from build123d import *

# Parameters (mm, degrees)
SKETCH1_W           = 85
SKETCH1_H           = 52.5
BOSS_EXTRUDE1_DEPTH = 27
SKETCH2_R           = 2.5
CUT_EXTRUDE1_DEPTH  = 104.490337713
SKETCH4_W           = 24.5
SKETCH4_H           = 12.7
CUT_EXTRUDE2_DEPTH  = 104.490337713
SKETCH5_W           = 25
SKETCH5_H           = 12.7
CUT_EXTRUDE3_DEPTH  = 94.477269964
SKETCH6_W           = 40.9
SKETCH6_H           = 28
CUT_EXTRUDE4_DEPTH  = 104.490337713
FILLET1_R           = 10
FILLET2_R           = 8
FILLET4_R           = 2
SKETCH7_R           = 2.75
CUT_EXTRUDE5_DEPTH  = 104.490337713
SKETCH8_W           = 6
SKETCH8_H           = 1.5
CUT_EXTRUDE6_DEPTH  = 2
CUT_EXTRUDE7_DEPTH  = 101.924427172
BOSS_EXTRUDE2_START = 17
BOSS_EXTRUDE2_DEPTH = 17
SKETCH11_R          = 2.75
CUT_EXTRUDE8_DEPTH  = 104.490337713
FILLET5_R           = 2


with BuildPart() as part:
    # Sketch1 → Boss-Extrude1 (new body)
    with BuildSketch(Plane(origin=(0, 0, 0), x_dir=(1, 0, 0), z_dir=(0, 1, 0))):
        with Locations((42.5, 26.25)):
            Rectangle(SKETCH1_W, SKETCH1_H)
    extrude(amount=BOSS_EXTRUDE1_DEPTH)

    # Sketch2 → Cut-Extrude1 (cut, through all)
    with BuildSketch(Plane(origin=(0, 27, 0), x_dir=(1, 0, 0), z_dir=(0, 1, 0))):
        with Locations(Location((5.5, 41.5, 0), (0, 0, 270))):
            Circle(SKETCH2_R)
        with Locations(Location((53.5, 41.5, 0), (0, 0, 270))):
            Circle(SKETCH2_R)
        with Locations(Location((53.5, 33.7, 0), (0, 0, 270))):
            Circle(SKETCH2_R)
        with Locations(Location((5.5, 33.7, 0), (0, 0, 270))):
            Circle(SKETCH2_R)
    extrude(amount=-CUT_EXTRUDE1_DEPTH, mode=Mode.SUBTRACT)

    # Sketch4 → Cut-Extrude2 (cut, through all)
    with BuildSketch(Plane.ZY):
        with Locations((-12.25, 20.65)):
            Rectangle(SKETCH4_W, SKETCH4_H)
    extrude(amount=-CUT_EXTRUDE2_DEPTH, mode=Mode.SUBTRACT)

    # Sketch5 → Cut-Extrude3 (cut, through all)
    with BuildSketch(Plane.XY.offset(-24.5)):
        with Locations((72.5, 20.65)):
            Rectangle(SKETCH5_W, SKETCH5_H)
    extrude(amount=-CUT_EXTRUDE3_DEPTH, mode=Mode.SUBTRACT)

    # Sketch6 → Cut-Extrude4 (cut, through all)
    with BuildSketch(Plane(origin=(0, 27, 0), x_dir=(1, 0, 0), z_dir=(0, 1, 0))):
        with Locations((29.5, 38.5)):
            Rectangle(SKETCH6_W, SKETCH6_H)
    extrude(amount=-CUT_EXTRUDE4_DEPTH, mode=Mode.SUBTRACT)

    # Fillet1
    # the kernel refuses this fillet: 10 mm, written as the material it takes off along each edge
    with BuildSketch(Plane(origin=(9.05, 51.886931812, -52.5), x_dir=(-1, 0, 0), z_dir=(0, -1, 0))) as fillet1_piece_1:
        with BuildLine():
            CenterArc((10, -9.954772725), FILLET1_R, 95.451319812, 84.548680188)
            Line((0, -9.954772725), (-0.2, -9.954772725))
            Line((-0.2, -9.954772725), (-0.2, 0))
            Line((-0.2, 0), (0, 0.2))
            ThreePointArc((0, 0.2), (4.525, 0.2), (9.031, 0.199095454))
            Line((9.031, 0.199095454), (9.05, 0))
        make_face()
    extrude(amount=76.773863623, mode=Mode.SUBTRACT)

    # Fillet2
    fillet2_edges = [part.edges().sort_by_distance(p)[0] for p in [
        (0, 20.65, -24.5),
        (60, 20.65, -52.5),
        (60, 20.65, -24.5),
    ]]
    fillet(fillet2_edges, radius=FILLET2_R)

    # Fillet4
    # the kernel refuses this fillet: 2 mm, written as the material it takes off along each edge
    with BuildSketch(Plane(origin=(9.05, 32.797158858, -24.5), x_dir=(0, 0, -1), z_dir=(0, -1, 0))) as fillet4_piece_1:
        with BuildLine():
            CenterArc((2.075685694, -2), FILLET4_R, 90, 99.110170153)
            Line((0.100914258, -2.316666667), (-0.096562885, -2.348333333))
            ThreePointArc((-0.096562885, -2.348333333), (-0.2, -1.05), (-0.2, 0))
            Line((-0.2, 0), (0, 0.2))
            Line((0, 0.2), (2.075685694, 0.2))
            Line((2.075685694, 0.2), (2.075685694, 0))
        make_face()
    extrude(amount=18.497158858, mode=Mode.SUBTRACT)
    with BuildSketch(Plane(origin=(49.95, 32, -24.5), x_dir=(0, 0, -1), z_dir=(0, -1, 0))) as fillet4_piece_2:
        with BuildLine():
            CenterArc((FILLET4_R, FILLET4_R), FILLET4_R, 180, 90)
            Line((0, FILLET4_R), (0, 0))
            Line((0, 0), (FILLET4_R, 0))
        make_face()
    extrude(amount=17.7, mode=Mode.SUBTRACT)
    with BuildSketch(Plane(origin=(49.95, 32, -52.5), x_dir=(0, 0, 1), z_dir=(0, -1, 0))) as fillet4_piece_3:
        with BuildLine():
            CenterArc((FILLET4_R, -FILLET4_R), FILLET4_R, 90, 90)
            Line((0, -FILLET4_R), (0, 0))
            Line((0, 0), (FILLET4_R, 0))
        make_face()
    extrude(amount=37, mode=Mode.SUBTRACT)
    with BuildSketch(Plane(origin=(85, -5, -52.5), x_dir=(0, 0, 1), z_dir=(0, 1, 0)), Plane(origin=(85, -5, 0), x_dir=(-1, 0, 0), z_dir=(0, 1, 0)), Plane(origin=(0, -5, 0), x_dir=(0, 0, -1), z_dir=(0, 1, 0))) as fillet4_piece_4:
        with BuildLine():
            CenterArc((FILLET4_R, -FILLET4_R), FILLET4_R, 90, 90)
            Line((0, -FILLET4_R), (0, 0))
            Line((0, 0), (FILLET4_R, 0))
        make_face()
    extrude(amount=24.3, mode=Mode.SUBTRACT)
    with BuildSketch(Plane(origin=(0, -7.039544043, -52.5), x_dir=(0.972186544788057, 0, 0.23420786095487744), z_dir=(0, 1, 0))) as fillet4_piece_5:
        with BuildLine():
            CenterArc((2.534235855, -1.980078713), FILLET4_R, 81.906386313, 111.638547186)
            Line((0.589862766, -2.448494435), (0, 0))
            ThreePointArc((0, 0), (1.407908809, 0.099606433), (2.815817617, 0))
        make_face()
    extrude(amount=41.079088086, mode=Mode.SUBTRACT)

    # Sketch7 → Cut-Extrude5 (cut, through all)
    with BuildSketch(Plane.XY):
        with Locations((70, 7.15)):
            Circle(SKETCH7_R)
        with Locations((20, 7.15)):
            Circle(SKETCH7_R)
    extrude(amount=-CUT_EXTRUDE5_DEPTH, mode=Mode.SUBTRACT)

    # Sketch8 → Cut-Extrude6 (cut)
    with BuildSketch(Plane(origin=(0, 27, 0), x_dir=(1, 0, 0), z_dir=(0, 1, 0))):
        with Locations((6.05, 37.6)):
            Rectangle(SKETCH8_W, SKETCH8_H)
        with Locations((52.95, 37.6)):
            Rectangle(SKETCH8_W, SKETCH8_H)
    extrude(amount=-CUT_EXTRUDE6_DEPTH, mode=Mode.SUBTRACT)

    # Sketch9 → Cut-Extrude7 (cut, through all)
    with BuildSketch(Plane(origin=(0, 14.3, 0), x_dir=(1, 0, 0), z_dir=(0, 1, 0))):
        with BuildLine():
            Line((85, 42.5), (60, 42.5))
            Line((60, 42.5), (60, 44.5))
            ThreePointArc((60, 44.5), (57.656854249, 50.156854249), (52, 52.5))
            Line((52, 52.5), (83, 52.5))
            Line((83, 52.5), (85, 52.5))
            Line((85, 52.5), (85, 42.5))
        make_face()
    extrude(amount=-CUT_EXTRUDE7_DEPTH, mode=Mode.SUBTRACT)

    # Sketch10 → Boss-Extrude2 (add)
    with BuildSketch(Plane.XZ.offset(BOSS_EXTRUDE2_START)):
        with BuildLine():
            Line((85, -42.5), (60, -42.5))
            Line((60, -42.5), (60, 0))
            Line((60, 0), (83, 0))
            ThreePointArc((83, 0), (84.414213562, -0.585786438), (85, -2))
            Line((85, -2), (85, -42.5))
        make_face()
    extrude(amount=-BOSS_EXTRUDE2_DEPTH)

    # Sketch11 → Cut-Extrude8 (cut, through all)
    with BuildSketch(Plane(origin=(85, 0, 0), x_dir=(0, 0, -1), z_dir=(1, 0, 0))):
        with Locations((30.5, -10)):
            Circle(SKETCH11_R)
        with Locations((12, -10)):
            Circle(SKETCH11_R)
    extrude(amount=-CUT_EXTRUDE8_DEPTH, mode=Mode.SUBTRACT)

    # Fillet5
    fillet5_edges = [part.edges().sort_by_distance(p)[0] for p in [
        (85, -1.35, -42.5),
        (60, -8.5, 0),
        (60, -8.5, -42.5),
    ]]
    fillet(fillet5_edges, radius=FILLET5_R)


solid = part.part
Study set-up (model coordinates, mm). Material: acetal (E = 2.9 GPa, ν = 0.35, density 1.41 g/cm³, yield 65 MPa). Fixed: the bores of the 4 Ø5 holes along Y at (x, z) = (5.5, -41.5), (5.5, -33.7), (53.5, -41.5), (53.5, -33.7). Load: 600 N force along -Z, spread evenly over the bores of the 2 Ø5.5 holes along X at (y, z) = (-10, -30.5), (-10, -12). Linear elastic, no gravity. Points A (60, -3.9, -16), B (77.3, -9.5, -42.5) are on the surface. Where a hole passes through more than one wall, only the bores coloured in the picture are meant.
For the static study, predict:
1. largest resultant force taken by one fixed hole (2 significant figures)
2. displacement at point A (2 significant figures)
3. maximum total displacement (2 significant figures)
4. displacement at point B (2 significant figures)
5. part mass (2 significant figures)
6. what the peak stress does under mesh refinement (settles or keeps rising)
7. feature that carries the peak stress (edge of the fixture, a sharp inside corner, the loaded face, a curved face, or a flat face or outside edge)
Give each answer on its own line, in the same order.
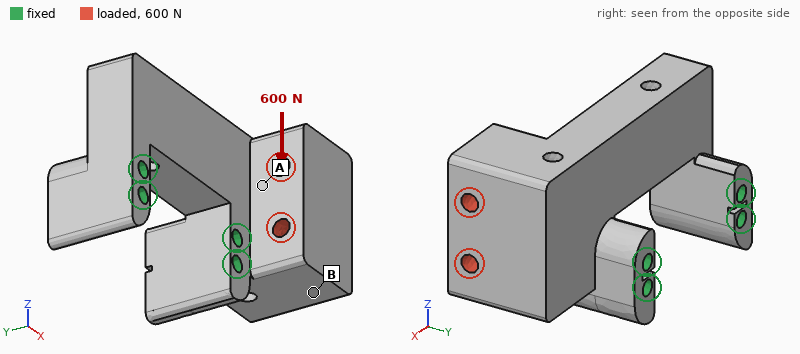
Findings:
610 N
0.11 mm
0.24 mm
0.14 mm
88 g
keeps rising
a sharp inside corner
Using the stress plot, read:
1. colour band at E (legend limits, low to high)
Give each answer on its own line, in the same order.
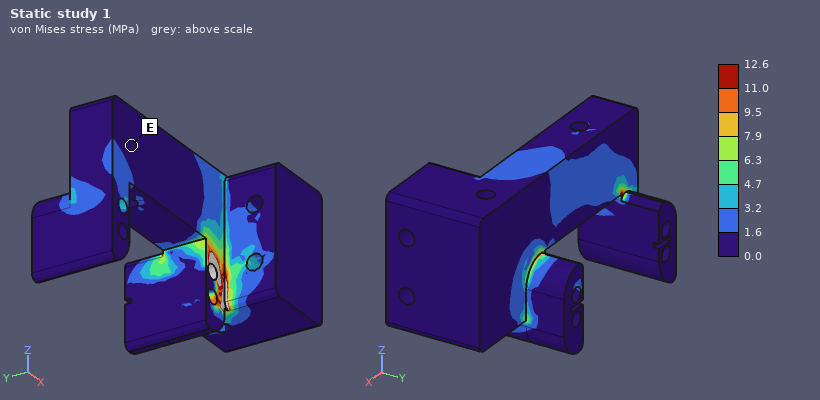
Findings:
0.0 to 1.6 MPa
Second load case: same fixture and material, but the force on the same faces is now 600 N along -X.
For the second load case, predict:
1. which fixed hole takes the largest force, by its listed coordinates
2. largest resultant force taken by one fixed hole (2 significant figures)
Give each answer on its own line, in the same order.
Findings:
(53.5, -33.7)
520 N
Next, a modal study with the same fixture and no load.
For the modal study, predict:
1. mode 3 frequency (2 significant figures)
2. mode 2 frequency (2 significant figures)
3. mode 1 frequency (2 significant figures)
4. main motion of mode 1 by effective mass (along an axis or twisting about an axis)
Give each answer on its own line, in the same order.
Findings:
2100 Hz
1600 Hz
1300 Hz
along Y
